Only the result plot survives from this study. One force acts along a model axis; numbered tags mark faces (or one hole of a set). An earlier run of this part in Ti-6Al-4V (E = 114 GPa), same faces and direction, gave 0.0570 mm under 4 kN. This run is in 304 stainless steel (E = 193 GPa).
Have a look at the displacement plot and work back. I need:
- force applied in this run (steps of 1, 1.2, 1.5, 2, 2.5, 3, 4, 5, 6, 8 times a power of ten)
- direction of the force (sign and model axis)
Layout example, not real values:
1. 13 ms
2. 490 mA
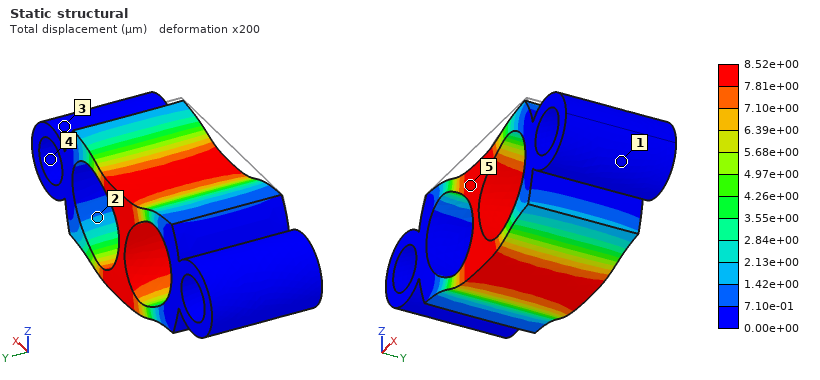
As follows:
1. 1 kN
2. -Z
